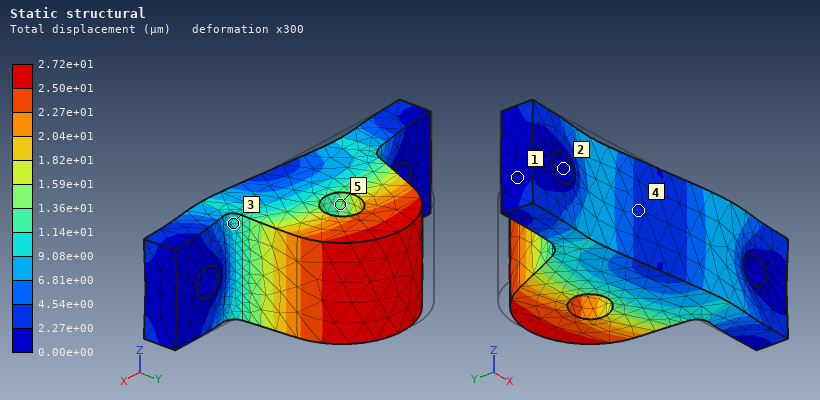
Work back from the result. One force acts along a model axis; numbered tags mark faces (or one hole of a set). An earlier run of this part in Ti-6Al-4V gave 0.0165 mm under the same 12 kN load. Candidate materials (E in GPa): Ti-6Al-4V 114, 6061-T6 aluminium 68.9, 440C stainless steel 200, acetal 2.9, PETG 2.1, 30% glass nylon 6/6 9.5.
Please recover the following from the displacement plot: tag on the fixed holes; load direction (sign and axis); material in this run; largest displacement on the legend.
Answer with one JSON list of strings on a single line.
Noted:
["2", "+X", "6061-T6 aluminium", "2.72e+01 µm"]
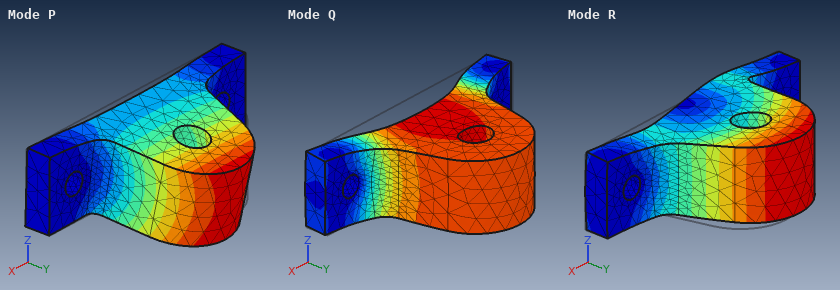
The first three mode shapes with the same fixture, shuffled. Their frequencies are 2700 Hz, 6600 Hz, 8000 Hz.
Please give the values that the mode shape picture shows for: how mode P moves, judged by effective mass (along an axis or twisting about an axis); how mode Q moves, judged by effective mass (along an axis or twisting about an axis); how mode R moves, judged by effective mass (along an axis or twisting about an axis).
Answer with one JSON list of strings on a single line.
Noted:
["along Z", "along Y", "along X"]
